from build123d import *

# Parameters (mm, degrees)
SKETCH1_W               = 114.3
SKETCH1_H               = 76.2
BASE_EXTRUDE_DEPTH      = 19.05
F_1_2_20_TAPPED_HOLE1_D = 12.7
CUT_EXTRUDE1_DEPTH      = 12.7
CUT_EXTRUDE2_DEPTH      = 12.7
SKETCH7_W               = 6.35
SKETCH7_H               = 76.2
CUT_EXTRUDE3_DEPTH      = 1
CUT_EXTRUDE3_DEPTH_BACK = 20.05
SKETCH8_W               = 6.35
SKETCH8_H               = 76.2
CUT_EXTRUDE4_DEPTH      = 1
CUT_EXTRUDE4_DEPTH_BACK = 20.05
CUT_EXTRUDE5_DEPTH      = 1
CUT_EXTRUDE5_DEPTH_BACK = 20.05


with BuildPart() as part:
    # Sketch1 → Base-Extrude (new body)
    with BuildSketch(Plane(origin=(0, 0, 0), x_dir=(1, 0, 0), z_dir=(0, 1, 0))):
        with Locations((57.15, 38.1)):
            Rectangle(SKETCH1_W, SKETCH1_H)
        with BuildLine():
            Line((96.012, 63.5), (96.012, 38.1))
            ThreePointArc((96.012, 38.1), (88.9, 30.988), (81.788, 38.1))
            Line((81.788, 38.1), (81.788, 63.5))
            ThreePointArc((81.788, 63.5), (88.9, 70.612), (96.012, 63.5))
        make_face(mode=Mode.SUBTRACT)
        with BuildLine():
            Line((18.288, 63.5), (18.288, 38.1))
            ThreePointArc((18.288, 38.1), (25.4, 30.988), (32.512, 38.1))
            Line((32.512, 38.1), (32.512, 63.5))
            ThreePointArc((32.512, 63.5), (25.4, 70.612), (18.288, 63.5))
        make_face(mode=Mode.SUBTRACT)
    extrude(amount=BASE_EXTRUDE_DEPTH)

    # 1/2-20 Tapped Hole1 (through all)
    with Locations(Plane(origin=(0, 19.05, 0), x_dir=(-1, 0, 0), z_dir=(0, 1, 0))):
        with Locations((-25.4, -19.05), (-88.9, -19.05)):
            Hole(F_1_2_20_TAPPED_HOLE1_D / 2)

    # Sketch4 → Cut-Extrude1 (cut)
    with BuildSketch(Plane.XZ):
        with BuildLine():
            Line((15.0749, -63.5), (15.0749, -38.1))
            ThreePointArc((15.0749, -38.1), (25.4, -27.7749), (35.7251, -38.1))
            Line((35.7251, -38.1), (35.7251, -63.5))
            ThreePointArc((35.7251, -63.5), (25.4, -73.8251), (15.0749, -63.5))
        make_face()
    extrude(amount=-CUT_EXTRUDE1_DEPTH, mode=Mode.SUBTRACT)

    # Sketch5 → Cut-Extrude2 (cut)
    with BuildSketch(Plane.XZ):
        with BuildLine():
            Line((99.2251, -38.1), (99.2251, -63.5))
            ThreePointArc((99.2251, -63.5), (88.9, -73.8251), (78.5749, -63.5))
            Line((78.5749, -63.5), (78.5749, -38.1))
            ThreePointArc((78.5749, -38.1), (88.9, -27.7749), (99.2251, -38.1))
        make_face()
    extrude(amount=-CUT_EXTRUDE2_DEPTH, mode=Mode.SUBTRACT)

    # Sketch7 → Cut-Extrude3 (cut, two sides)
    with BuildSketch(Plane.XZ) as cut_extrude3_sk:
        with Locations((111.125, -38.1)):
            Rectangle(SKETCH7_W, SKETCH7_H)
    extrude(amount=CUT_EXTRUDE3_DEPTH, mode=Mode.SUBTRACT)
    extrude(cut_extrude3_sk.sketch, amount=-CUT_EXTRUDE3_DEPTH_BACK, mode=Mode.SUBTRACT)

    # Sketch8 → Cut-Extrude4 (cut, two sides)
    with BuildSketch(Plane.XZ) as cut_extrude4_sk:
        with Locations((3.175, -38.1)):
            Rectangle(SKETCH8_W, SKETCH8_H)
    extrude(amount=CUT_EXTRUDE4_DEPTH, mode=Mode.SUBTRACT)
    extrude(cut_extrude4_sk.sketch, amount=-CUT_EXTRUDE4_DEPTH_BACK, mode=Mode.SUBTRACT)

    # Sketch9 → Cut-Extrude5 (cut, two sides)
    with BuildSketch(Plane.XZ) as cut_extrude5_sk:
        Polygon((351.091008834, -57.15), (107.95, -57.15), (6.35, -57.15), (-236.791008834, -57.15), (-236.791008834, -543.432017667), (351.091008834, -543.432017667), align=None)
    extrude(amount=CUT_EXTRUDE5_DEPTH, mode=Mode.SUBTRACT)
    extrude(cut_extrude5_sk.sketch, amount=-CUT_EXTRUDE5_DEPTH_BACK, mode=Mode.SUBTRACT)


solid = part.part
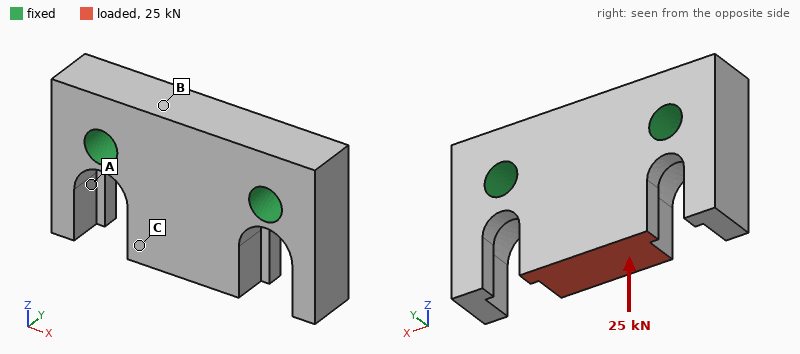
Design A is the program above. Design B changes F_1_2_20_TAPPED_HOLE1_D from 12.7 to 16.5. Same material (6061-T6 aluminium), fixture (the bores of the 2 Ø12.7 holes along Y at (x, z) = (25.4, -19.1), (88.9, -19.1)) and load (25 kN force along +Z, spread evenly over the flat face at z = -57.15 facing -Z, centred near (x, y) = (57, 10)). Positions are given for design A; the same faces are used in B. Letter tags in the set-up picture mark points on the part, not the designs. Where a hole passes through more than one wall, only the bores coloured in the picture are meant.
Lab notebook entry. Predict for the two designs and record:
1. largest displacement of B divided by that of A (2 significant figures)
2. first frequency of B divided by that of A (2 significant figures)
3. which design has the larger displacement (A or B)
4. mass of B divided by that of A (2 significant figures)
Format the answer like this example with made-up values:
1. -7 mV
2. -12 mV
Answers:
1. 0.89
2. 1.1
3. A
4. 0.96
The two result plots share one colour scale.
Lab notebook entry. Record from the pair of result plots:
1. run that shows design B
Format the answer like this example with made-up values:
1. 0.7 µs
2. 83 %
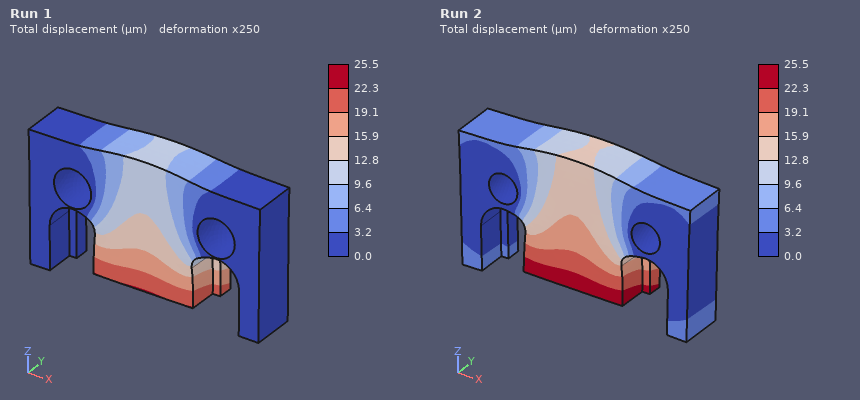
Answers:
1. Run 1
